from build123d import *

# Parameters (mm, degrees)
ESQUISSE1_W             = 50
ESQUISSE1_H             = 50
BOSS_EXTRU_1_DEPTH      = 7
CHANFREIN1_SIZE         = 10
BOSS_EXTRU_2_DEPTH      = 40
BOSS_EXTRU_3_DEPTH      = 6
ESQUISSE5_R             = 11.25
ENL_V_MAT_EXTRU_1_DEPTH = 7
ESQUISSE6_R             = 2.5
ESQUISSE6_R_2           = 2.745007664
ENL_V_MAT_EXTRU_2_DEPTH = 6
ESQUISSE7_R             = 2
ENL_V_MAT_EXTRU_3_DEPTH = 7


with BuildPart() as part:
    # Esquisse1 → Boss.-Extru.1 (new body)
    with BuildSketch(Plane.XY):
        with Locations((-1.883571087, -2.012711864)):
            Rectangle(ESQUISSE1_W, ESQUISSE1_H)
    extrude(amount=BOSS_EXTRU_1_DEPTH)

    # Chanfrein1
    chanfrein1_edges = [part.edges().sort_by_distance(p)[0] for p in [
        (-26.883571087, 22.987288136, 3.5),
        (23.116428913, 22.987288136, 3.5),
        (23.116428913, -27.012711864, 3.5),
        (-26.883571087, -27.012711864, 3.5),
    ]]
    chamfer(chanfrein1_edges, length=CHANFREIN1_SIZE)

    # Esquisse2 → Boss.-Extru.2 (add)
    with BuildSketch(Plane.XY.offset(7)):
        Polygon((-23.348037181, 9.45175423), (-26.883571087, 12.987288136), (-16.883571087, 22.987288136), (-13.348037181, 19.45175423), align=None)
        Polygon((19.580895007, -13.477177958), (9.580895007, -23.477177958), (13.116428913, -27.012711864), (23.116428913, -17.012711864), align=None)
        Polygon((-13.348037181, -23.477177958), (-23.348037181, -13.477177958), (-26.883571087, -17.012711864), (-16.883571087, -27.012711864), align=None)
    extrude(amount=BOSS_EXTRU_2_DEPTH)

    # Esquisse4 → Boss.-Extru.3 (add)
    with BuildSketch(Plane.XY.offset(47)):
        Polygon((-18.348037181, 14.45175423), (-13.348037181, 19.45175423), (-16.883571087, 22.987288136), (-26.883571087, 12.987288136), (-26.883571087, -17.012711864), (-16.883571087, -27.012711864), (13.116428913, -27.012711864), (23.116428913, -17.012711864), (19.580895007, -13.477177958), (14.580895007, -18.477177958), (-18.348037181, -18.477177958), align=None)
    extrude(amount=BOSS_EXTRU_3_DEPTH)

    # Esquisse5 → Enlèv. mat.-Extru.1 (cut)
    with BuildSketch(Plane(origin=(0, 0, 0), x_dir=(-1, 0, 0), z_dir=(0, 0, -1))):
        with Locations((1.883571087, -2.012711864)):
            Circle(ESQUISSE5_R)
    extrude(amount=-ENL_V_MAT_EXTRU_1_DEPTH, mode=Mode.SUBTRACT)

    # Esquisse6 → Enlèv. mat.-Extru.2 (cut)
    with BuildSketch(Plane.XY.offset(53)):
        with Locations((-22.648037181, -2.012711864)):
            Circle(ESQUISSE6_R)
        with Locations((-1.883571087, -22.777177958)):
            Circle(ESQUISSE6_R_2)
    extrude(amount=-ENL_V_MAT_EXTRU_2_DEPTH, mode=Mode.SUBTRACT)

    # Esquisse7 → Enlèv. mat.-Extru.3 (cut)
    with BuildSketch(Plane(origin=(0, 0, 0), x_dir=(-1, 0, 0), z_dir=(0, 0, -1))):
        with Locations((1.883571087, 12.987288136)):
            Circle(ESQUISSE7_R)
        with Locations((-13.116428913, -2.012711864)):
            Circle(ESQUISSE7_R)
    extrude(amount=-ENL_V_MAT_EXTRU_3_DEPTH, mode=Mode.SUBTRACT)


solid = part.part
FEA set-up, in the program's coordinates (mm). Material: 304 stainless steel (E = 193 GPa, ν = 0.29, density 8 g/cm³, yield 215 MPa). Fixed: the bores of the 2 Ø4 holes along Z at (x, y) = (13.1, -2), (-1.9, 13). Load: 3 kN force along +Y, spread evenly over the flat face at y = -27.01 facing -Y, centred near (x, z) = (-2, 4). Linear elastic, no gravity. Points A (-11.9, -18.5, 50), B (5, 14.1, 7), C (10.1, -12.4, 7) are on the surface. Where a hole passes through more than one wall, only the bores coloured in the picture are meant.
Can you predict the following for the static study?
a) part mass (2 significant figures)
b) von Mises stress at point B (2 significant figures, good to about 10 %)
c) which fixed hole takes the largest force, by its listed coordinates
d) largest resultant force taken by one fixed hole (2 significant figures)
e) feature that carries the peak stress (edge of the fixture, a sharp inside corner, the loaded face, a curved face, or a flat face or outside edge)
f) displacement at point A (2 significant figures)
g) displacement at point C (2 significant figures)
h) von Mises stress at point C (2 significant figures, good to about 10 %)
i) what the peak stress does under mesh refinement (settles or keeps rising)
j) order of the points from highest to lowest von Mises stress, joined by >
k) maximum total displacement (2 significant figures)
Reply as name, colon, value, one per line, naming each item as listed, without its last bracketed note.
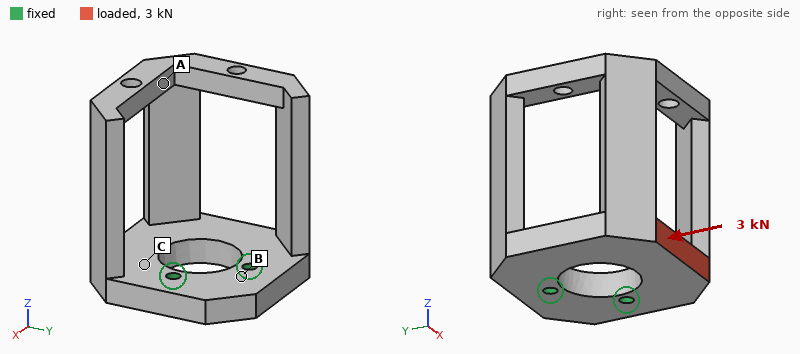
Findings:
part mass: 200 g
von Mises stress at point B: 16 MPa
which fixed hole takes the largest force, by its listed coordinates: (-1.9, 13)
largest resultant force taken by one fixed hole: 1.8 kN
feature that carries the peak stress: edge of the fixture
displacement at point A: 12 µm
displacement at point C: 5.0 µm
von Mises stress at point C: 33 MPa
what the peak stress does under mesh refinement: keeps rising
order of the points from highest to lowest von Mises stress, joined by >: C > B > A
maximum total displacement: 15 µm
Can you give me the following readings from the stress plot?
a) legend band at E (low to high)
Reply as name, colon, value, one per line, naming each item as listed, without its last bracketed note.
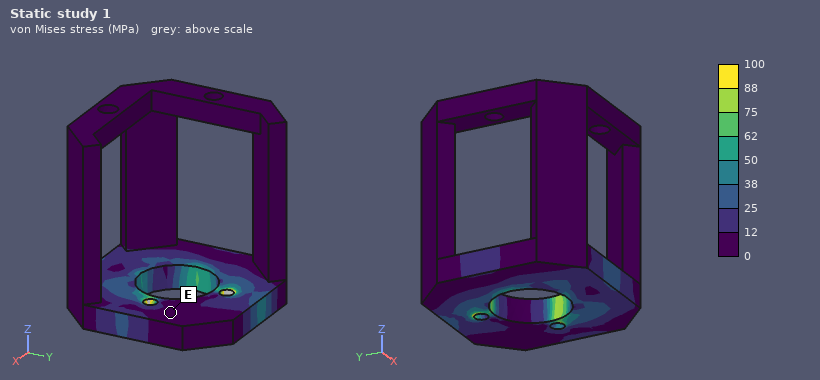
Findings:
legend band at E: 0 to 12 MPa
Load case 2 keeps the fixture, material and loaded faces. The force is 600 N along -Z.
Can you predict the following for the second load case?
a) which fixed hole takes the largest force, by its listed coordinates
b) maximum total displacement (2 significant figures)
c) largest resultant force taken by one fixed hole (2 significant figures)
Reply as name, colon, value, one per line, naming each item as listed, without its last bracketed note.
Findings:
which fixed hole takes the largest force, by its listed coordinates: (13.1, -2)
maximum total displacement: 78 µm
largest resultant force taken by one fixed hole: 540 N
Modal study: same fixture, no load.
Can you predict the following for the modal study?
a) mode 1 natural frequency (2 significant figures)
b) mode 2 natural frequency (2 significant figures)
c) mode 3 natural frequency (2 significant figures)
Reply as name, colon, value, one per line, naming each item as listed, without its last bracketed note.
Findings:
mode 1 natural frequency: 1300 Hz
mode 2 natural frequency: 1500 Hz
mode 3 natural frequency: 3300 Hz
